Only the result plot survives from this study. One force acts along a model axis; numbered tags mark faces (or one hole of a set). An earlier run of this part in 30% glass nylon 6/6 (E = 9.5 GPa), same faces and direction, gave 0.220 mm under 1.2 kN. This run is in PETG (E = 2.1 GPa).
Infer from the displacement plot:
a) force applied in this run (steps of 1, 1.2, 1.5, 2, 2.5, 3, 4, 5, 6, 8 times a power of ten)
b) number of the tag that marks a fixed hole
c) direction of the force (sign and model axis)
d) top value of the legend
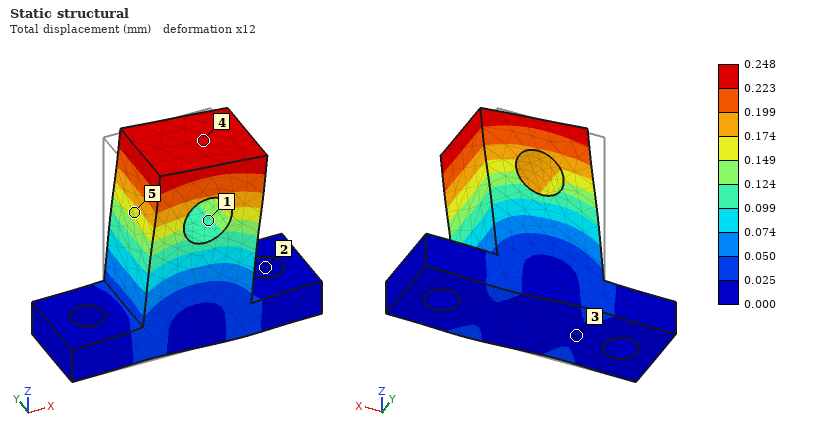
300 N
2
+X
0.248 mm
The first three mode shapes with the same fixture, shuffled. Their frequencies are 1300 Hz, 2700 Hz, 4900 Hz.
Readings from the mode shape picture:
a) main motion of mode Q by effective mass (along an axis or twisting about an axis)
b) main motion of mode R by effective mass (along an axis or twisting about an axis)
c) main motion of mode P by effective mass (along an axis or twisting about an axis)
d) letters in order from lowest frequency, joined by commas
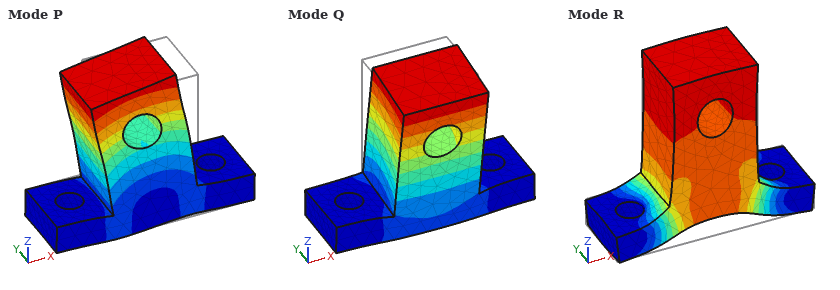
along Y
along Z
along X
Q, P, R
